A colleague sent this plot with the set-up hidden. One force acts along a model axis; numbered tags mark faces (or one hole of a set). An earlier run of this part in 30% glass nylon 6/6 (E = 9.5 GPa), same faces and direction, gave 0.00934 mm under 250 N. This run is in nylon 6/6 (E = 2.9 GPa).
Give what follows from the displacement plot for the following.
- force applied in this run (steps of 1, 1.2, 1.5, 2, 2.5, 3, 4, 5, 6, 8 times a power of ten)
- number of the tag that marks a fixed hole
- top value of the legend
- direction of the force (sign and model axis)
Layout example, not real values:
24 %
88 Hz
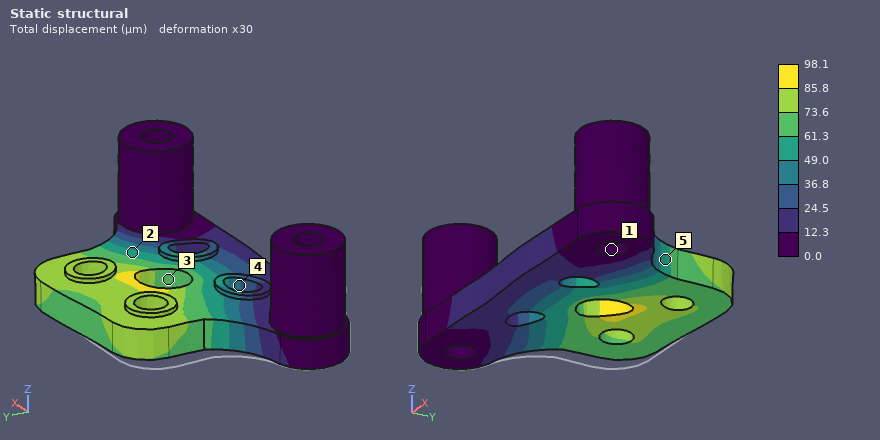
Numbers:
800 N
1
98.1 µm
+X
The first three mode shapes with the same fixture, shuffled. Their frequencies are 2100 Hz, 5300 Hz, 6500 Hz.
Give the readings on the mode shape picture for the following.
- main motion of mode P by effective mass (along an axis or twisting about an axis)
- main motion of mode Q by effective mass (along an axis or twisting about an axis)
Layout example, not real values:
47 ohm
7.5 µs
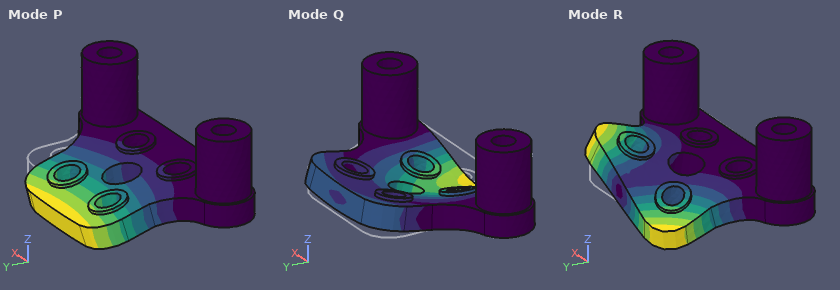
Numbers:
along Z
along Z
